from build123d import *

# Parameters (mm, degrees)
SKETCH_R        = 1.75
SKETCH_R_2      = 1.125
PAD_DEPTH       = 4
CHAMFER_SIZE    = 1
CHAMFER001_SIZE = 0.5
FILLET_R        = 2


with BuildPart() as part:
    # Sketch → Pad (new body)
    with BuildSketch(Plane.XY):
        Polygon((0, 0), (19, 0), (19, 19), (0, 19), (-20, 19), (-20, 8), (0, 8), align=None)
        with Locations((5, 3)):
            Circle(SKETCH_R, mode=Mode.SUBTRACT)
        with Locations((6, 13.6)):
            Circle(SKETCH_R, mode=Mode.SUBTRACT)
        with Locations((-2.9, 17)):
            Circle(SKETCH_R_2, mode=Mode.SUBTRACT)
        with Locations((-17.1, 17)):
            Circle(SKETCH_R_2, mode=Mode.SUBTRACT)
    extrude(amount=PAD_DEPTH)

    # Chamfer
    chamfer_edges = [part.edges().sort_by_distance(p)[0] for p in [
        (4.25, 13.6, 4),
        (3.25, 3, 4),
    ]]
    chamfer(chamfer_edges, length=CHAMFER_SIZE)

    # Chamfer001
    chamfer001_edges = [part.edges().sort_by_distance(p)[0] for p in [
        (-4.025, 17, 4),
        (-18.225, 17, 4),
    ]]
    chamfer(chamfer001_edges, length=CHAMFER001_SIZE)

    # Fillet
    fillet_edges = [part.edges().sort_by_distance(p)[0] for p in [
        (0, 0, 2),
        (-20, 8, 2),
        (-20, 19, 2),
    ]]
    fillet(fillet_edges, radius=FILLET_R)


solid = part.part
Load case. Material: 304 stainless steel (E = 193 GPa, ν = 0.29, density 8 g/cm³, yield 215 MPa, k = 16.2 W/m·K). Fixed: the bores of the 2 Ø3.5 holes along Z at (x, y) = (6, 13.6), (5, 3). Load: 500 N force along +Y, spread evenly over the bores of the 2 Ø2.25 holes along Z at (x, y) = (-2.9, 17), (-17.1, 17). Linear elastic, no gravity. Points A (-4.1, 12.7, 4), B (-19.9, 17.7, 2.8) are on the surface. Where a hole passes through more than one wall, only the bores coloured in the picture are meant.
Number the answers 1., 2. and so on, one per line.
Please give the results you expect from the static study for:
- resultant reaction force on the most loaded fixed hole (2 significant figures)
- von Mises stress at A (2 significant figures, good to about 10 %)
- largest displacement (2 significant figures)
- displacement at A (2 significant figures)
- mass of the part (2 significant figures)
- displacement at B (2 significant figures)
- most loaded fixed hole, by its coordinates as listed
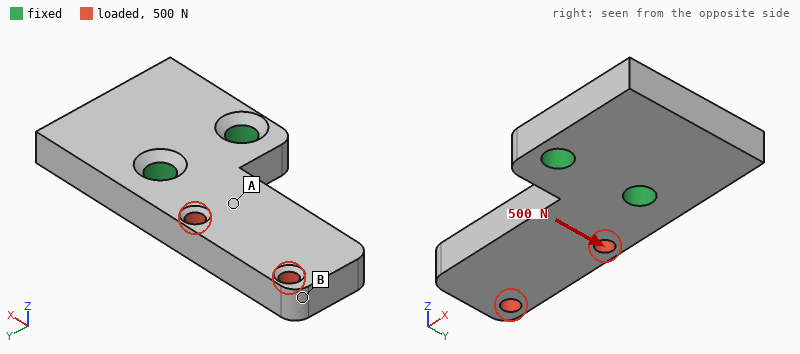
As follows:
1. 680 N
2. 22 MPa
3. 19 µm
4. 3.9 µm
5. 18 g
6. 19 µm
7. (5, 3)
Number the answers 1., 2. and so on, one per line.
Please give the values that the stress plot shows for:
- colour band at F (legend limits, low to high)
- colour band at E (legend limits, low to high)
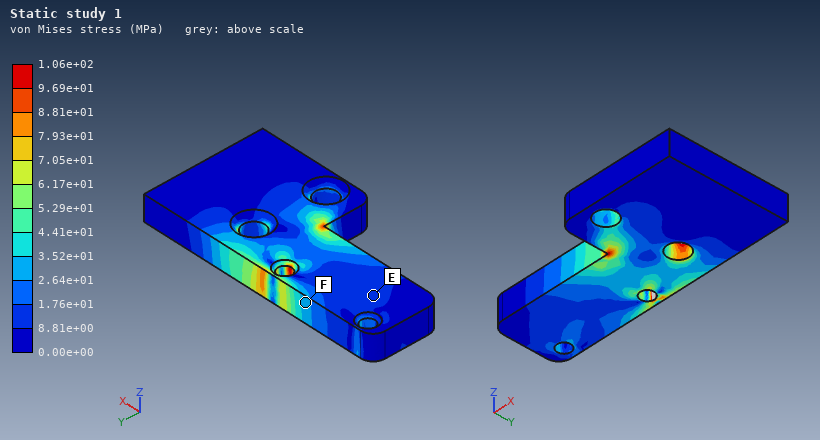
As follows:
1. 2.64e+01 to 3.52e+01 MPa
2. 8.81e+00 to 1.76e+01 MPa
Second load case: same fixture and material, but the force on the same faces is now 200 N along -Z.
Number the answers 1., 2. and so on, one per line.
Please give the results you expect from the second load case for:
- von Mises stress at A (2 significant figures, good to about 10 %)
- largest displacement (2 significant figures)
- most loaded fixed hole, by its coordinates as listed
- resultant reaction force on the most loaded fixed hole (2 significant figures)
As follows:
1. 53 MPa
2. 54 µm
3. (6, 13.6)
4. 210 N
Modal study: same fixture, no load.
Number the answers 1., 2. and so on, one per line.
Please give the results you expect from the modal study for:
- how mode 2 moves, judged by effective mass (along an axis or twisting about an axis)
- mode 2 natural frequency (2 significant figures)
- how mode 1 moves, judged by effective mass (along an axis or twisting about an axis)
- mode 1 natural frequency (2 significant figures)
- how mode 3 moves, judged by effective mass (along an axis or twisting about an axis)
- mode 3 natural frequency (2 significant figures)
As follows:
1. along Y
2. 12 kHz
3. along Z
4. 4900 Hz
5. along Z
6. 16 kHz
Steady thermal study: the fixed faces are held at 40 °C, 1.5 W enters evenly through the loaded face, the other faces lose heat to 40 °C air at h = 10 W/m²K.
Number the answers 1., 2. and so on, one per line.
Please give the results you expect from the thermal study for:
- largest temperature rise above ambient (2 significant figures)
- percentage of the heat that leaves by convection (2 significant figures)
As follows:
1. 35 K
2. 10 %
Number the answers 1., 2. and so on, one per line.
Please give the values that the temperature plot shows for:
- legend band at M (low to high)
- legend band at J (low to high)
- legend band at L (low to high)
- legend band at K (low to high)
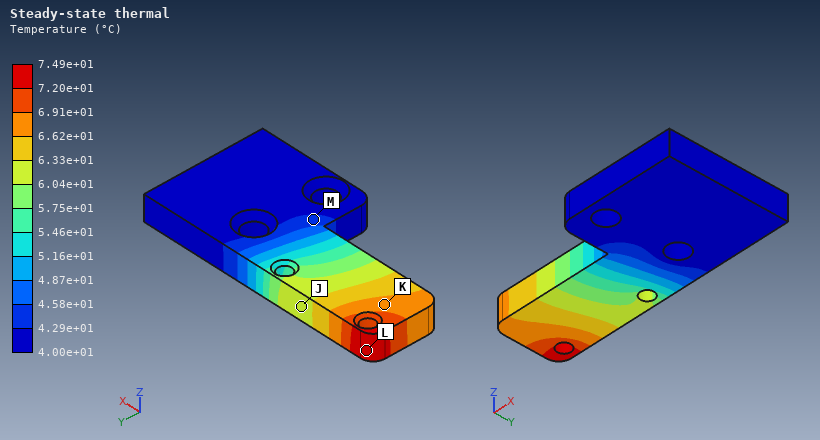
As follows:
1. 4.29e+01 to 4.58e+01 °C
2. 6.04e+01 to 6.33e+01 °C
3. 7.20e+01 to 7.49e+01 °C
4. 6.62e+01 to 6.91e+01 °C
